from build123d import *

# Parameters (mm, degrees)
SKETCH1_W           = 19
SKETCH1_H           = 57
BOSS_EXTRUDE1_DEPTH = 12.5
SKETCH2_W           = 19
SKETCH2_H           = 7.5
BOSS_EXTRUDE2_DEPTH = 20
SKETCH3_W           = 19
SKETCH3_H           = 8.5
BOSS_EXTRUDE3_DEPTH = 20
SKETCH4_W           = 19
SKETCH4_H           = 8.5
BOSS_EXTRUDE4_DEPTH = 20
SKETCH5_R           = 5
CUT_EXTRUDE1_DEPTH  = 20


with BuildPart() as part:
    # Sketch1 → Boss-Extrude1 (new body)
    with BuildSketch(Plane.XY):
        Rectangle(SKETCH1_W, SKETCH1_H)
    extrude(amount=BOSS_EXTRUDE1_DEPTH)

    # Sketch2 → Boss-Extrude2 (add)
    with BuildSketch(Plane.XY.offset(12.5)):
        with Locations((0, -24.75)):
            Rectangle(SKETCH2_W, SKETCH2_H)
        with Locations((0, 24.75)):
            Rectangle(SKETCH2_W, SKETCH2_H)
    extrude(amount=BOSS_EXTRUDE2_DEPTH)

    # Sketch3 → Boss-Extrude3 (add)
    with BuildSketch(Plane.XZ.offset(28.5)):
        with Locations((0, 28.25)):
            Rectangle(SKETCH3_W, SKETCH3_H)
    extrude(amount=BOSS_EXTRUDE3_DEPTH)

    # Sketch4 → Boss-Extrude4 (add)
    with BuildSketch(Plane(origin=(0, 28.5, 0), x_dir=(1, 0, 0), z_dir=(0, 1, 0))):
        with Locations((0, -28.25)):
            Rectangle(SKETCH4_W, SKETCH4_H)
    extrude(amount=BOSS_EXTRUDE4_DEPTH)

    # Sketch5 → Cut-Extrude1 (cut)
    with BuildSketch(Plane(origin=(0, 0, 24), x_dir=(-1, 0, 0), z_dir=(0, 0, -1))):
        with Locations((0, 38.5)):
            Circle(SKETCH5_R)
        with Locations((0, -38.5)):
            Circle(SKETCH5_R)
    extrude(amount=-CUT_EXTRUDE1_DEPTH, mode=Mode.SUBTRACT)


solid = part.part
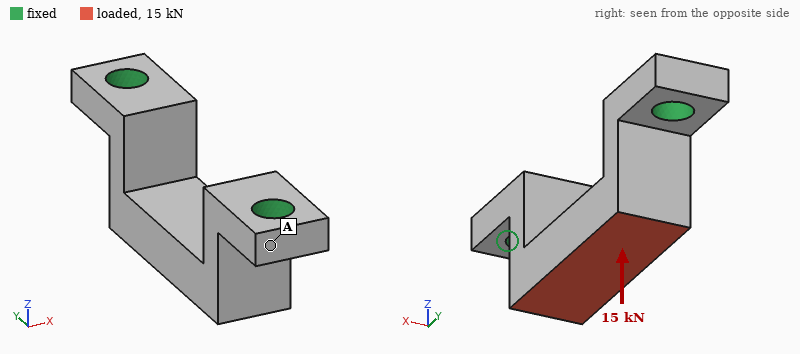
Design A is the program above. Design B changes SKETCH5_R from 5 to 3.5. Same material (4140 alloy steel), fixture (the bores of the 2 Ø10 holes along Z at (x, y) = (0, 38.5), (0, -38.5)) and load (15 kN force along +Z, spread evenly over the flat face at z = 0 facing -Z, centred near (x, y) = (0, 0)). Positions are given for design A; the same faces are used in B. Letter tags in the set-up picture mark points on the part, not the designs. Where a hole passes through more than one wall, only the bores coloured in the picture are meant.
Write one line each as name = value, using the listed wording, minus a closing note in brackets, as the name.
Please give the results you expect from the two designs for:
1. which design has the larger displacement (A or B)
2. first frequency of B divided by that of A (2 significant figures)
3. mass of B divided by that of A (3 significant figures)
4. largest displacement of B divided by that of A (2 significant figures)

which design has the larger displacement = B
first frequency of B divided by that of A = 0.89
mass of B divided by that of A = 1.03
largest displacement of B divided by that of A = 1.1
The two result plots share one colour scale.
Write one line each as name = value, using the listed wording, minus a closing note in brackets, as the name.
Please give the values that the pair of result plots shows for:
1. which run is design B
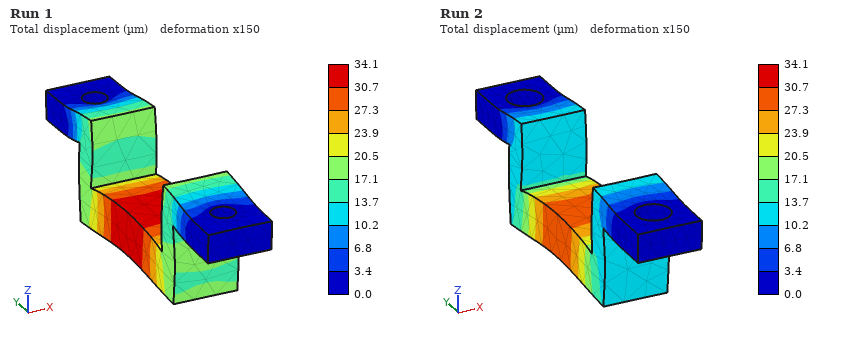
which run is design B = Run 1
